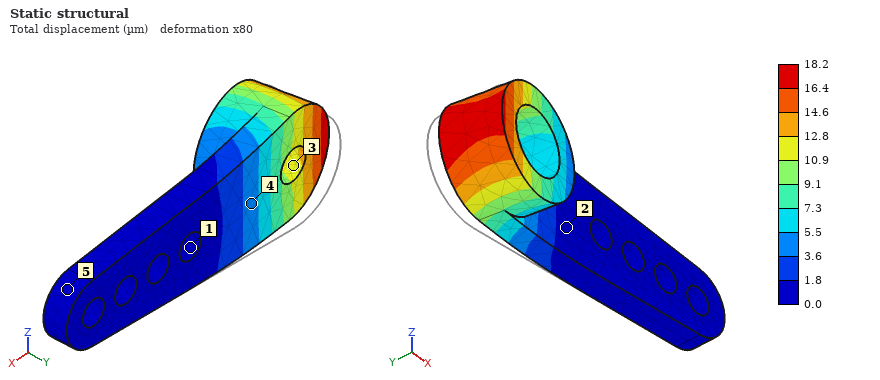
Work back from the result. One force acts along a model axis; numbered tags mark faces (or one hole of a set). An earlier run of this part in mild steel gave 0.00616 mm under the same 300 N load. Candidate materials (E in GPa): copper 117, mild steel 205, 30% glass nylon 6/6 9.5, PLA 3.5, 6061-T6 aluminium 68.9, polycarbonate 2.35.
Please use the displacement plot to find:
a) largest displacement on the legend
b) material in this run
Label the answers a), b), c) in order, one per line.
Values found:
a) 18.2 µm
b) 6061-T6 aluminium
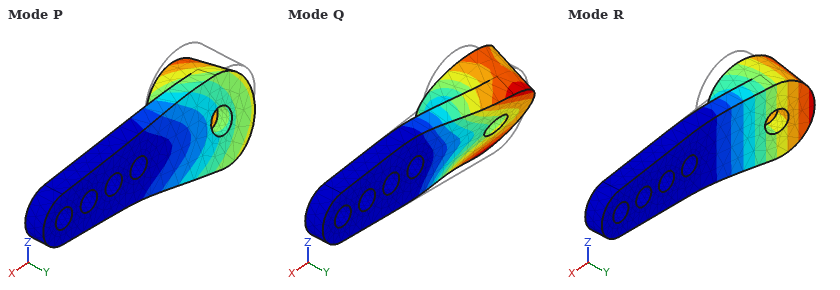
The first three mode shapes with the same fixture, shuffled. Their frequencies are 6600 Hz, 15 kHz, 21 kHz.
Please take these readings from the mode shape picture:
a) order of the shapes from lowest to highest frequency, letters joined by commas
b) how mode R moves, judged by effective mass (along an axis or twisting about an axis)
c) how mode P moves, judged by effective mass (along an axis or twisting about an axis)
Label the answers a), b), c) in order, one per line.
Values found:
a) R, P, Q
b) along Y
c) along Z
